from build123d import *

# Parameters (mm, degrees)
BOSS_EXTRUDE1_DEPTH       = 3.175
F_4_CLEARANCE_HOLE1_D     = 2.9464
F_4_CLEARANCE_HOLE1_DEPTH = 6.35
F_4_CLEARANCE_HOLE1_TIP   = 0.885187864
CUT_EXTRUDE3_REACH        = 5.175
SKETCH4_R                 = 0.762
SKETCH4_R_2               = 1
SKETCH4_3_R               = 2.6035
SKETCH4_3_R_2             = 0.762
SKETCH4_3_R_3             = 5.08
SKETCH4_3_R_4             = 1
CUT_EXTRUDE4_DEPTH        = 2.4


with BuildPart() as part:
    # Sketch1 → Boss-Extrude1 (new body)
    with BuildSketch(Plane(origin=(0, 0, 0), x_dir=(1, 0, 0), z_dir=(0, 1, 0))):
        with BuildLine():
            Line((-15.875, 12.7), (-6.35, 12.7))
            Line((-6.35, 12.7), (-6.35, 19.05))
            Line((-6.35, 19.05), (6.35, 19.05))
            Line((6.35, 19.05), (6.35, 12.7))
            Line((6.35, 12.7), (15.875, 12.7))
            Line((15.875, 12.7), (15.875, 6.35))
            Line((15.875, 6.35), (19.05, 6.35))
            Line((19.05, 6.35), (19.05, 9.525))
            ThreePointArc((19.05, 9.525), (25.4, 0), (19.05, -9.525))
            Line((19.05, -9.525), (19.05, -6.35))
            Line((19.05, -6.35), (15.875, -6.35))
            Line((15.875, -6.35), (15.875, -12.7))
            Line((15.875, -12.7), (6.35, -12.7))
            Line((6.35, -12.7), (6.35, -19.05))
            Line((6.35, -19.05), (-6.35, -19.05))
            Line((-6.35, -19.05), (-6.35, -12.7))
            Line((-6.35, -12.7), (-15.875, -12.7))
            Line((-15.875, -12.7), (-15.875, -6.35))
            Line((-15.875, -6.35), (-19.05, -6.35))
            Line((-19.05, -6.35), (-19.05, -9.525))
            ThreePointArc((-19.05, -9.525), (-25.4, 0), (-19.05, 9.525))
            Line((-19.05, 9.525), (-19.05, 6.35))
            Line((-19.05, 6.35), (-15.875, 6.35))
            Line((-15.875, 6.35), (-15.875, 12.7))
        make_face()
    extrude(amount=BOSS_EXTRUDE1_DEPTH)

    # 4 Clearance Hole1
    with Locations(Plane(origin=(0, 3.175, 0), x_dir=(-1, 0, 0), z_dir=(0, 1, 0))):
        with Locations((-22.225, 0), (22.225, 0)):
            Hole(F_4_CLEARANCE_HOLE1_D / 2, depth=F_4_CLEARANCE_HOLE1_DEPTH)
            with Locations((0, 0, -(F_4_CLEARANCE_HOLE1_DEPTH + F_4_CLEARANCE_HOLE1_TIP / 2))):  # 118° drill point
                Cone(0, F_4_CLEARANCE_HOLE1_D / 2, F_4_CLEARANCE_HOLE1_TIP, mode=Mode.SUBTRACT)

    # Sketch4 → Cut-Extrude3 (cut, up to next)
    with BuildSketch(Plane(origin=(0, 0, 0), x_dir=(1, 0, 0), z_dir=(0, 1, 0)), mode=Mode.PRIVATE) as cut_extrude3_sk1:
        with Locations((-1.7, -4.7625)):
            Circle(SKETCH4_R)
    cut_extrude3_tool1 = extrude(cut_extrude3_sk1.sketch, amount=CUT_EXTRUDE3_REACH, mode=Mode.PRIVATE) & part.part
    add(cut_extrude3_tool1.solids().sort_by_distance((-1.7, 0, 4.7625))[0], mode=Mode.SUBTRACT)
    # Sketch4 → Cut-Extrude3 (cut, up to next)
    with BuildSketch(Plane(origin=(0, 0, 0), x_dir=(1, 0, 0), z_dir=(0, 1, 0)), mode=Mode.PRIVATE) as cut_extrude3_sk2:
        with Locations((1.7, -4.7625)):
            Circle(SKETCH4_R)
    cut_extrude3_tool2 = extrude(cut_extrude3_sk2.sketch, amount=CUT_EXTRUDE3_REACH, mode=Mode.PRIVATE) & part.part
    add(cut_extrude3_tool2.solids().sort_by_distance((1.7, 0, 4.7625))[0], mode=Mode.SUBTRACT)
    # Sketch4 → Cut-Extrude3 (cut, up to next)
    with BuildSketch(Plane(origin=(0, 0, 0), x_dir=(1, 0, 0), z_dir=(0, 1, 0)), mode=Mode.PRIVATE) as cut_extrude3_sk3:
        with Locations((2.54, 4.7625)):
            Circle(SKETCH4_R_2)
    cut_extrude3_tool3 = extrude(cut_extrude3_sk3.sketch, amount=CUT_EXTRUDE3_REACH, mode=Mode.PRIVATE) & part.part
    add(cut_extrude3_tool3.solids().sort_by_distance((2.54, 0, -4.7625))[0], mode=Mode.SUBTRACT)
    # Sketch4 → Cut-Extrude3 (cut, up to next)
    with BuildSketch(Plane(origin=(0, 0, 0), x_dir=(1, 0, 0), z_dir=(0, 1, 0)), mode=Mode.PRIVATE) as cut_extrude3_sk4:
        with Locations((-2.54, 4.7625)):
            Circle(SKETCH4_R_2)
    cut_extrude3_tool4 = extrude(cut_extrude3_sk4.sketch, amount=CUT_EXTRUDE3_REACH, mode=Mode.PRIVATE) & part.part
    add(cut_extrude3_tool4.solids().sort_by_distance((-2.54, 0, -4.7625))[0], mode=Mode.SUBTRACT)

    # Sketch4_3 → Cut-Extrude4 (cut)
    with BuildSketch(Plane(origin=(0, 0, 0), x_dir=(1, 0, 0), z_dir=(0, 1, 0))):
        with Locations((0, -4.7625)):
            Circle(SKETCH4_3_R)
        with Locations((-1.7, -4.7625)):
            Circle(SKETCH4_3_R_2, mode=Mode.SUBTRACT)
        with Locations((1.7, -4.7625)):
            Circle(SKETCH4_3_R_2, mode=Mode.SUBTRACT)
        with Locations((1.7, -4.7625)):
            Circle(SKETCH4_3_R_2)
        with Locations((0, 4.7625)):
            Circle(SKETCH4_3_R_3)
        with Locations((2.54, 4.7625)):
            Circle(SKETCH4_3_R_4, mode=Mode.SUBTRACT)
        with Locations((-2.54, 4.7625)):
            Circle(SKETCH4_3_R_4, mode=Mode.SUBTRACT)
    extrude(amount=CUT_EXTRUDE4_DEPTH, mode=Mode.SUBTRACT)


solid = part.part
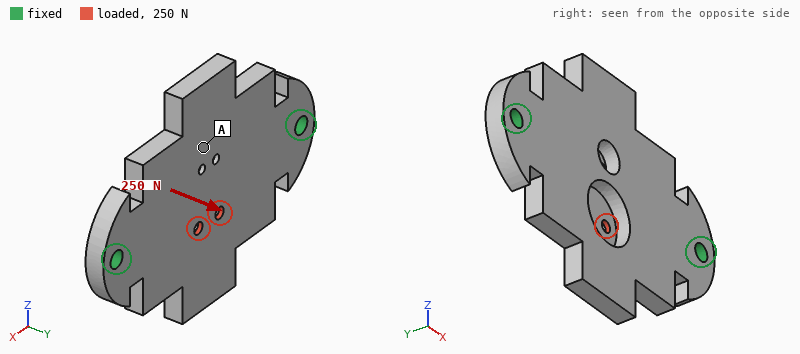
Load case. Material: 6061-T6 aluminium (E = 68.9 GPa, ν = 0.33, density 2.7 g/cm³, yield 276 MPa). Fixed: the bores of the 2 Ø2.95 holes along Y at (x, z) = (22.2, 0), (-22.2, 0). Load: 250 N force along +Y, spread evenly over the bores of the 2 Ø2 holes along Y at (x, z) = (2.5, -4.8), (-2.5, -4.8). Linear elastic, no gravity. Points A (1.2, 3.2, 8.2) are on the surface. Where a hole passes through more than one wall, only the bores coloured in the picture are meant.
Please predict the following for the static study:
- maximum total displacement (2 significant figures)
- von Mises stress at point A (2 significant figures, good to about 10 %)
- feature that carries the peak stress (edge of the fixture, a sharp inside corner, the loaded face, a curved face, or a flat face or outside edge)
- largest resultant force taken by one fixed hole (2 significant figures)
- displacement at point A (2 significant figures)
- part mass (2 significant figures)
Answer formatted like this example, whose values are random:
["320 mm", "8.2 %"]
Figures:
["83 µm", "19 MPa", "the loaded face", "150 N", "18 µm", "9.7 g"]
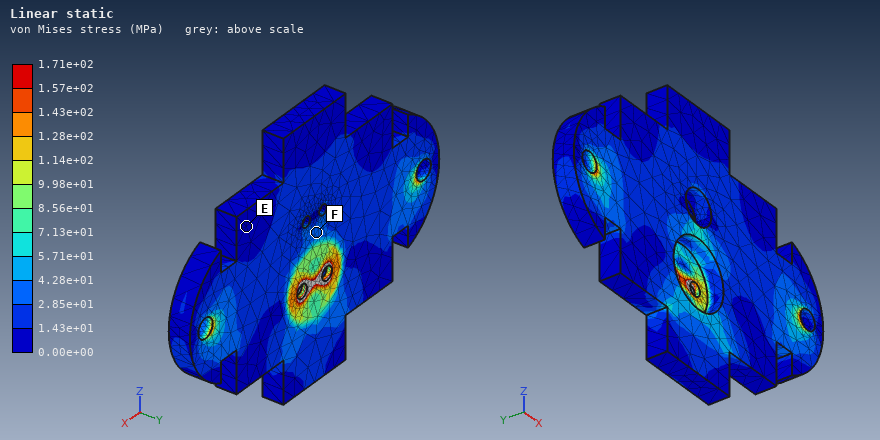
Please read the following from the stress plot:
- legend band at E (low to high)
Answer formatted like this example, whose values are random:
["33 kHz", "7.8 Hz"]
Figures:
["0.00e+00 to 1.43e+01 MPa"]
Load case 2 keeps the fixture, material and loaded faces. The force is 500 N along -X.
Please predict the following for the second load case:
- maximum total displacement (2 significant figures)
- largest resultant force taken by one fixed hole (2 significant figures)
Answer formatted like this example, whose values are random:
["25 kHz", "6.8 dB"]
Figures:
["6.5 µm", "260 N"]
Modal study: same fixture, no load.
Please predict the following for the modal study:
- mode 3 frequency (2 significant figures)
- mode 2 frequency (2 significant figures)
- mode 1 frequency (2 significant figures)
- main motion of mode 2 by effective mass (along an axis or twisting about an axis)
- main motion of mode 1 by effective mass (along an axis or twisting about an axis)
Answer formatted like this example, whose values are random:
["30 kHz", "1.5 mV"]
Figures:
["15 kHz", "5400 Hz", "4500 Hz", "along Y", "twisting about X"]
